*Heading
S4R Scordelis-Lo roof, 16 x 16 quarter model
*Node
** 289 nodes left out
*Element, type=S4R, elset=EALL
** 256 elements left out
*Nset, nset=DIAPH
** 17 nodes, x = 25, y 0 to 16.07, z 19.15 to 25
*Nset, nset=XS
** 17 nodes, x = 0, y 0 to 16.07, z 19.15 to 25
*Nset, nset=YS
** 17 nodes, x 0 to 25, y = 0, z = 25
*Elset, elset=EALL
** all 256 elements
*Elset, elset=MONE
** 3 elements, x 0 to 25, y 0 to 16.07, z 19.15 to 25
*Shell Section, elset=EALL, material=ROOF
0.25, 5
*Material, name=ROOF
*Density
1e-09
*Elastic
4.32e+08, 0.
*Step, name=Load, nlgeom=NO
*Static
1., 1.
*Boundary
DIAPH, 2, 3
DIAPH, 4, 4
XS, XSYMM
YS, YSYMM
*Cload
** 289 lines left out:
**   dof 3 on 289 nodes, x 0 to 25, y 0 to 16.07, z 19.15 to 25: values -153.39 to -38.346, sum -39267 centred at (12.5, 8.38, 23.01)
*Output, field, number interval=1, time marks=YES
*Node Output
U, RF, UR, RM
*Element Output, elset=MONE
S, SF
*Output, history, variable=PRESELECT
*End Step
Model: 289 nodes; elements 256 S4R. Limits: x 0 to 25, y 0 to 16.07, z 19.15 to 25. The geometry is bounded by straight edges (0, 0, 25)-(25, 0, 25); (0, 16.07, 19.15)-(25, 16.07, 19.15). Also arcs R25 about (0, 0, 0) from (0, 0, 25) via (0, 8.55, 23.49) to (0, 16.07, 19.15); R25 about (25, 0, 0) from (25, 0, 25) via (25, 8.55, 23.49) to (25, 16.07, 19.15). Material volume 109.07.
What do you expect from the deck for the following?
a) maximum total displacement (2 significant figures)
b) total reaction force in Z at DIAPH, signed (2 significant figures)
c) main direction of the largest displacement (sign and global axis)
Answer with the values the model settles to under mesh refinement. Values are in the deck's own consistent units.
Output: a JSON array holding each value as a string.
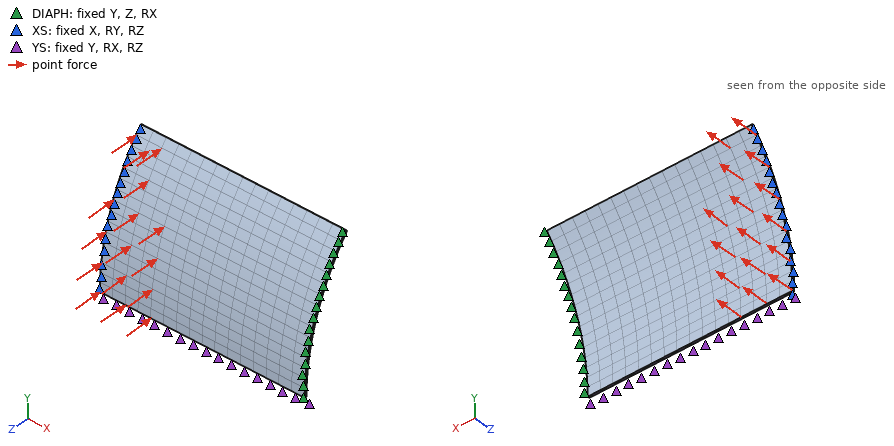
["0.070", "39000", "-Z"]
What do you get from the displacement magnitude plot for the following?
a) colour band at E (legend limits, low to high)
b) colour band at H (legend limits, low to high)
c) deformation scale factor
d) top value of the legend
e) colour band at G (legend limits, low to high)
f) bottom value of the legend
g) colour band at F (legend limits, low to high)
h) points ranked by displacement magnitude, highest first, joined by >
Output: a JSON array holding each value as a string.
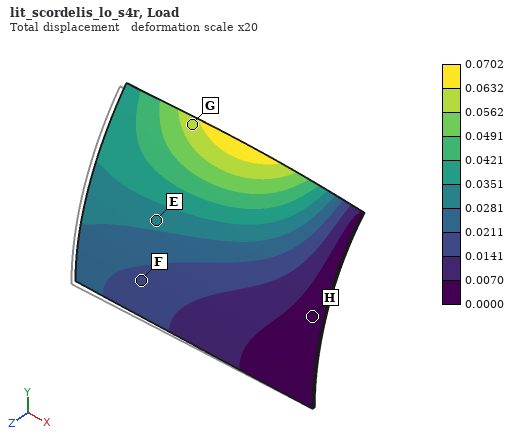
["0.0281 to 0.0351", "0.0000 to 0.0070", "20", "0.0702", "0.0562 to 0.0632", "0.0000", "0.0141 to 0.0211", "G > E > F > H"]
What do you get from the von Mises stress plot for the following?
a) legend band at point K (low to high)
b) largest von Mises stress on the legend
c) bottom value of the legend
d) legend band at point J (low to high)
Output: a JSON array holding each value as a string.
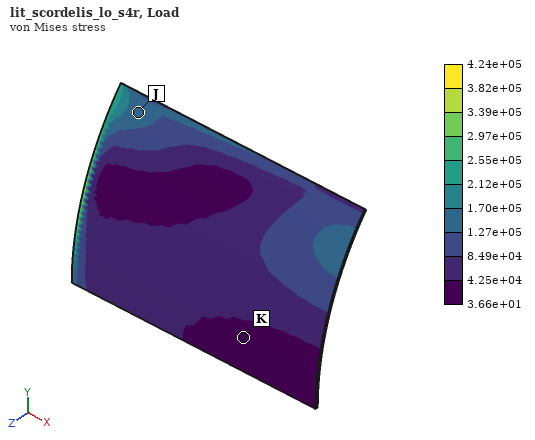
["3.66e+01 to 4.25e+04", "4.24e+05", "3.66e+01", "1.27e+05 to 1.70e+05"]
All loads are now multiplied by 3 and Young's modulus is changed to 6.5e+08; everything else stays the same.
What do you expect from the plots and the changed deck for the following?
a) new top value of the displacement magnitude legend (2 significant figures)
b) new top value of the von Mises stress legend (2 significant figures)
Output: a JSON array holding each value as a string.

["0.14", "1.3e+06"]
